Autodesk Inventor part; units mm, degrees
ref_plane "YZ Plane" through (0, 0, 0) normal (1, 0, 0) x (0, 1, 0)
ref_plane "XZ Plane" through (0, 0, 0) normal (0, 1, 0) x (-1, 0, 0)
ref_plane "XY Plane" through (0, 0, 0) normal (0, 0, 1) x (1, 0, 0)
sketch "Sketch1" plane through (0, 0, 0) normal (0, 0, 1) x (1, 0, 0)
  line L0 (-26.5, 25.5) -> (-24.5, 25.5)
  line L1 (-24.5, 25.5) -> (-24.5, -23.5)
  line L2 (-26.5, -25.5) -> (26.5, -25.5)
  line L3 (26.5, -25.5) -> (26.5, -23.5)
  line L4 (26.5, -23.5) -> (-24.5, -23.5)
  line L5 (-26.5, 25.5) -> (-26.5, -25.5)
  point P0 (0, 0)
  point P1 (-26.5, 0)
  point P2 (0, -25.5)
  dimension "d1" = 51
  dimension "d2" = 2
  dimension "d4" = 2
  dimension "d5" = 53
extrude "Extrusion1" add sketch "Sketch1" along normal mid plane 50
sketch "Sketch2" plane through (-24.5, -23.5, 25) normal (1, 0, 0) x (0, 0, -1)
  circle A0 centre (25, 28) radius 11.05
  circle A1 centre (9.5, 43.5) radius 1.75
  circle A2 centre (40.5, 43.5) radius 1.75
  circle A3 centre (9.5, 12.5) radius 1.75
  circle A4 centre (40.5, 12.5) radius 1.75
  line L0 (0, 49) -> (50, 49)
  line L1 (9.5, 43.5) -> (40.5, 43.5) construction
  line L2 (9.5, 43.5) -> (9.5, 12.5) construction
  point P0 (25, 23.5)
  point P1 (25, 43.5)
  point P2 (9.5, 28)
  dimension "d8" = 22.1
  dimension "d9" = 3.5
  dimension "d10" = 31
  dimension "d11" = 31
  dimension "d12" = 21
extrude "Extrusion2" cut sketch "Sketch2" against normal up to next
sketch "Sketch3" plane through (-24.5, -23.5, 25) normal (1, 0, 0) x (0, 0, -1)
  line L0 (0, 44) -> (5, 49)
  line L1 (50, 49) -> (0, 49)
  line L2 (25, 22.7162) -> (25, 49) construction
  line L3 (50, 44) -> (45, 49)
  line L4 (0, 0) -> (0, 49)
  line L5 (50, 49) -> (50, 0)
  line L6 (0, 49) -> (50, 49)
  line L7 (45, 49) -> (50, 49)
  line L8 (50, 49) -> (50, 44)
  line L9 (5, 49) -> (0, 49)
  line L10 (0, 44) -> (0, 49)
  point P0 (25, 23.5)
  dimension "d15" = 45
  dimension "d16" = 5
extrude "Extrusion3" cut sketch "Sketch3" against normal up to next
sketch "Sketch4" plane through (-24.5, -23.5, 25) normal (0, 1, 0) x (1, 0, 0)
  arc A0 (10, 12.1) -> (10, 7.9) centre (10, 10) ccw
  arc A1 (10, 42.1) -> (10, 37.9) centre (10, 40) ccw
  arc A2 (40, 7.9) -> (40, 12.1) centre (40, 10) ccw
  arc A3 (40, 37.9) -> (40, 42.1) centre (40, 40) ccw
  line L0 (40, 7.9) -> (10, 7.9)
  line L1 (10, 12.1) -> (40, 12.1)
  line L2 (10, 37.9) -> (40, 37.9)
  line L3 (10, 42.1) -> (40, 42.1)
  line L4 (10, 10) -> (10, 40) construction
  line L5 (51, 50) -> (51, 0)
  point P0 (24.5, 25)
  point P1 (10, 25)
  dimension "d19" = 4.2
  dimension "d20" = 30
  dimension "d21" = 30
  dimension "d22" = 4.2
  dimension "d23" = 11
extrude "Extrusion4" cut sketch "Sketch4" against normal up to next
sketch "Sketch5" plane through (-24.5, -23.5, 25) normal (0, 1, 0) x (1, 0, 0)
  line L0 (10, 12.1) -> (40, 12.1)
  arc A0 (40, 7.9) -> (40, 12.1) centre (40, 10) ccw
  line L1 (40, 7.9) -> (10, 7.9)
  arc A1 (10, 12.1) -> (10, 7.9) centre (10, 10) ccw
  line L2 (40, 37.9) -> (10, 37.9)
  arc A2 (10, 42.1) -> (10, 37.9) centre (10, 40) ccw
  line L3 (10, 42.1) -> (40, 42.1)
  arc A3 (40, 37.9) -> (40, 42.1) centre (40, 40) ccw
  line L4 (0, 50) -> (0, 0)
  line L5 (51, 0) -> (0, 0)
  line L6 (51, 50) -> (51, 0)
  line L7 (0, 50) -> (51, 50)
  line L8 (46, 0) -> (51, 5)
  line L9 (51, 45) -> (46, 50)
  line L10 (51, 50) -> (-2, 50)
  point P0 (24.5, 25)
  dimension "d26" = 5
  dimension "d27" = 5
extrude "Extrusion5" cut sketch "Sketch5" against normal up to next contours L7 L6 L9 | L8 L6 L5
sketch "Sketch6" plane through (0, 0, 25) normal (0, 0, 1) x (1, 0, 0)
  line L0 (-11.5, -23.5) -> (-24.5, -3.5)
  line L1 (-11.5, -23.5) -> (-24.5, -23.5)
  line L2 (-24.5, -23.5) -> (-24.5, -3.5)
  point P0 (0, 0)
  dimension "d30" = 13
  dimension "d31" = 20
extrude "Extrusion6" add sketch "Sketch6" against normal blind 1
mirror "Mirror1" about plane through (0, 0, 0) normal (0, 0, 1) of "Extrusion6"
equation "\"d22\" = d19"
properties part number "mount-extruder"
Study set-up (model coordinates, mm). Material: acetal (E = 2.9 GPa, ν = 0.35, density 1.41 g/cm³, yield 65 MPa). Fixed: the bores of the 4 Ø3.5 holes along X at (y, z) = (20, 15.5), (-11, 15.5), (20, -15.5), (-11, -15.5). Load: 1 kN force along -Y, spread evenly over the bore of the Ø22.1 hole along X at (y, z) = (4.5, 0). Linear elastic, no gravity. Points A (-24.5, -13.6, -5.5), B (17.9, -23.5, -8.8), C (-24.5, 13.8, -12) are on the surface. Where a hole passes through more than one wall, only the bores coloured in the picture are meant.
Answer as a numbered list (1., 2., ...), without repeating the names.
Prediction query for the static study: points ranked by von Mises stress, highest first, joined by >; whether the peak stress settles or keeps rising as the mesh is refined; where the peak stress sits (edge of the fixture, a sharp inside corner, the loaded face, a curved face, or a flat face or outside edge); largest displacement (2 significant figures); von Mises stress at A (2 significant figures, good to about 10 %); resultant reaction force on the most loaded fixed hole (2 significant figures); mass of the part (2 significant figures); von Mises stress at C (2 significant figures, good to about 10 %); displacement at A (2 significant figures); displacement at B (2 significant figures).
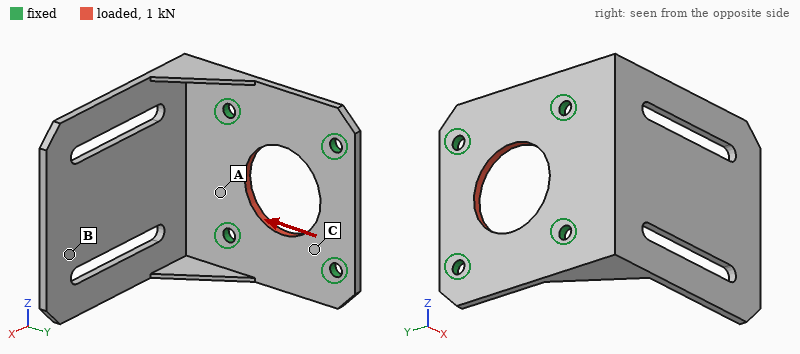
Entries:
1. C > A > B
2. keeps rising
3. edge of the fixture
4. 0.11 mm
5. 5.3 MPa
6. 260 N
7. 13 g
8. 11 MPa
9. 0.042 mm
10. 0.054 mm
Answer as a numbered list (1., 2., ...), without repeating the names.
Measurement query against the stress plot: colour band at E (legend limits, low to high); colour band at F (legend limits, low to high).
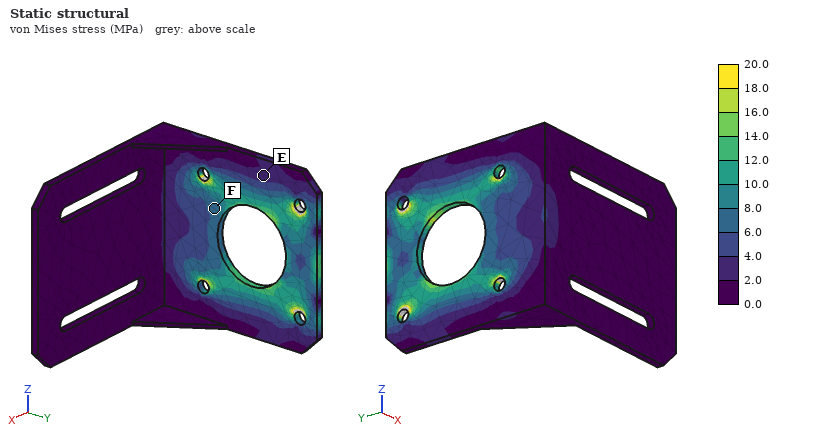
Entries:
1. 2.0 to 4.0 MPa
2. 6.0 to 8.0 MPa
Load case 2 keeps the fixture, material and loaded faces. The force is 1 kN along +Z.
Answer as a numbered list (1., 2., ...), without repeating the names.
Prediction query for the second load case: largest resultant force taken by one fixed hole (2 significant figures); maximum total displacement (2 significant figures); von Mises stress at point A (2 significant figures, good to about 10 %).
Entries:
1. 260 N
2. 83 µm
3. 4.7 MPa
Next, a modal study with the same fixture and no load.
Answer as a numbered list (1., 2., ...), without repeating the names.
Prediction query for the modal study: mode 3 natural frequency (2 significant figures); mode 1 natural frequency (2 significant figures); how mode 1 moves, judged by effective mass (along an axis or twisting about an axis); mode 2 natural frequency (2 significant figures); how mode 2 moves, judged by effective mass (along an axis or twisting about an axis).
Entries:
1. 610 Hz
2. 170 Hz
3. along Y
4. 400 Hz
5. along Z
